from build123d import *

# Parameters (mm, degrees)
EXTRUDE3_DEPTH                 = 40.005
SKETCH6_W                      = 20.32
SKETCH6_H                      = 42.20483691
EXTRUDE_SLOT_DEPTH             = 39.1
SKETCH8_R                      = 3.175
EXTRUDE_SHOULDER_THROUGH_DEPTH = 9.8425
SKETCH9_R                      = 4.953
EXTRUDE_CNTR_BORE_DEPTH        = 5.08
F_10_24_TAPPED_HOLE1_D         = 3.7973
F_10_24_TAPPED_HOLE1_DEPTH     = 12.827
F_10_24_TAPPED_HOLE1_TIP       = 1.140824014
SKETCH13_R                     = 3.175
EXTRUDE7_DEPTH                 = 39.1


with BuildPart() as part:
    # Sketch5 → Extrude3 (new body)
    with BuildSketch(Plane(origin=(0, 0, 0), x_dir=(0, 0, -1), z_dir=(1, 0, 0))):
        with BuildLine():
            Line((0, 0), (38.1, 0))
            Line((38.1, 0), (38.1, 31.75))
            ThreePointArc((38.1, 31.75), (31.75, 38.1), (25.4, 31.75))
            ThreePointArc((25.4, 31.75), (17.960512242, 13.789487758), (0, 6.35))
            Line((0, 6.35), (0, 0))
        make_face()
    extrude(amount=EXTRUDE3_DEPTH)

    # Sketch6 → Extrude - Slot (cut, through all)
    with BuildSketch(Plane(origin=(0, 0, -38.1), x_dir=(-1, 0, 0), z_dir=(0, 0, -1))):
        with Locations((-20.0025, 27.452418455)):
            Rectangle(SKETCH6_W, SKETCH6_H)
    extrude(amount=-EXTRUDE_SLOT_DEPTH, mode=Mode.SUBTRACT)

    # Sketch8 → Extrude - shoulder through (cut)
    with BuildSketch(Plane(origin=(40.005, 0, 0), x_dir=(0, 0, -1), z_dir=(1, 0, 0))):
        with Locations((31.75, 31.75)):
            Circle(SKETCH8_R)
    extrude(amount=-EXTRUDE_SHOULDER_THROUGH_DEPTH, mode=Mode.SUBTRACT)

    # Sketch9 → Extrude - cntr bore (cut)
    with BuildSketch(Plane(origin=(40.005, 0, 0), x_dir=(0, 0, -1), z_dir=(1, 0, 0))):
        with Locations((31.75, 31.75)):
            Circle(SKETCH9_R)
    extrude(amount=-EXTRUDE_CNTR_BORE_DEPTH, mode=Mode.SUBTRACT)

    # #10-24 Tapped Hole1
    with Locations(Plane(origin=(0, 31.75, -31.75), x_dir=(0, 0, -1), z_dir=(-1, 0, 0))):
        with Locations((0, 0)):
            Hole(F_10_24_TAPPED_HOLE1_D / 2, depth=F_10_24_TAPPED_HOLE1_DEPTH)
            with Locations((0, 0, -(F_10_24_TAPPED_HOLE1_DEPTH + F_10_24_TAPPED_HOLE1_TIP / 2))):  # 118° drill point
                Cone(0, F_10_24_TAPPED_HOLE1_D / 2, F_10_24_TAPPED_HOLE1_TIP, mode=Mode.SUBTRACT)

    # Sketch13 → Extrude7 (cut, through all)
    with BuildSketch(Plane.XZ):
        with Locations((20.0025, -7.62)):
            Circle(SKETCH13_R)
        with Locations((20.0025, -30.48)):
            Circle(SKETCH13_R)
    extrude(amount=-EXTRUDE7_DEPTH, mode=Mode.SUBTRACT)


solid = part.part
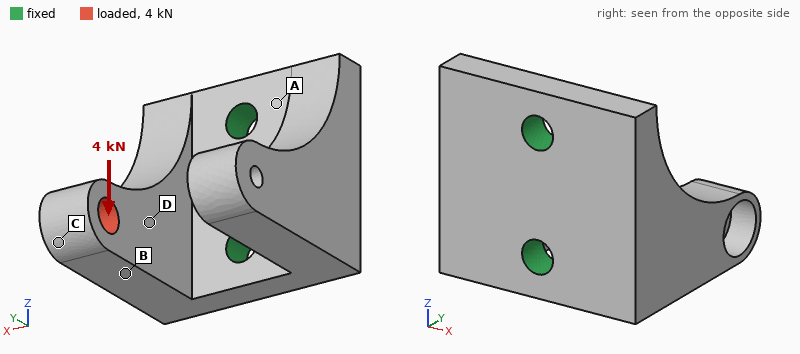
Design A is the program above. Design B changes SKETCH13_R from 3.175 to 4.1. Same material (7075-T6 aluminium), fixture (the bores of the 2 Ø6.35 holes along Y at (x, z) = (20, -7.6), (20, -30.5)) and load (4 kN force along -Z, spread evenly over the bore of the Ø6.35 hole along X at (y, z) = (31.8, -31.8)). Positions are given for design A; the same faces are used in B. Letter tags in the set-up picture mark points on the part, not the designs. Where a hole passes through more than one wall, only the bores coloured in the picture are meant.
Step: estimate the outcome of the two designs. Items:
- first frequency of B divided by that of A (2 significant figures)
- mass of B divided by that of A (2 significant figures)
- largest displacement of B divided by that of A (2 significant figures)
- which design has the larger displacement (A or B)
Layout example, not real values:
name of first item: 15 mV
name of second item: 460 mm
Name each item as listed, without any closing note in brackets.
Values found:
first frequency of B divided by that of A: 1.1
mass of B divided by that of A: 0.99
largest displacement of B divided by that of A: 0.92
which design has the larger displacement: A
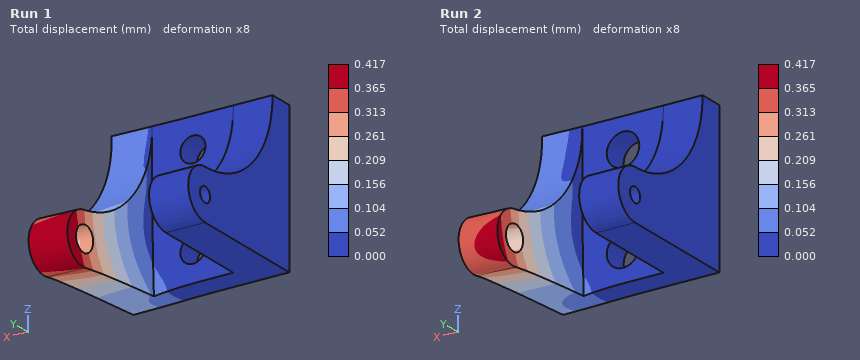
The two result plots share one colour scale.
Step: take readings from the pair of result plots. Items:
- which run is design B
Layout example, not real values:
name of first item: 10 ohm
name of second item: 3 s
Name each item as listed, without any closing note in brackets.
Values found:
which run is design B: Run 2
